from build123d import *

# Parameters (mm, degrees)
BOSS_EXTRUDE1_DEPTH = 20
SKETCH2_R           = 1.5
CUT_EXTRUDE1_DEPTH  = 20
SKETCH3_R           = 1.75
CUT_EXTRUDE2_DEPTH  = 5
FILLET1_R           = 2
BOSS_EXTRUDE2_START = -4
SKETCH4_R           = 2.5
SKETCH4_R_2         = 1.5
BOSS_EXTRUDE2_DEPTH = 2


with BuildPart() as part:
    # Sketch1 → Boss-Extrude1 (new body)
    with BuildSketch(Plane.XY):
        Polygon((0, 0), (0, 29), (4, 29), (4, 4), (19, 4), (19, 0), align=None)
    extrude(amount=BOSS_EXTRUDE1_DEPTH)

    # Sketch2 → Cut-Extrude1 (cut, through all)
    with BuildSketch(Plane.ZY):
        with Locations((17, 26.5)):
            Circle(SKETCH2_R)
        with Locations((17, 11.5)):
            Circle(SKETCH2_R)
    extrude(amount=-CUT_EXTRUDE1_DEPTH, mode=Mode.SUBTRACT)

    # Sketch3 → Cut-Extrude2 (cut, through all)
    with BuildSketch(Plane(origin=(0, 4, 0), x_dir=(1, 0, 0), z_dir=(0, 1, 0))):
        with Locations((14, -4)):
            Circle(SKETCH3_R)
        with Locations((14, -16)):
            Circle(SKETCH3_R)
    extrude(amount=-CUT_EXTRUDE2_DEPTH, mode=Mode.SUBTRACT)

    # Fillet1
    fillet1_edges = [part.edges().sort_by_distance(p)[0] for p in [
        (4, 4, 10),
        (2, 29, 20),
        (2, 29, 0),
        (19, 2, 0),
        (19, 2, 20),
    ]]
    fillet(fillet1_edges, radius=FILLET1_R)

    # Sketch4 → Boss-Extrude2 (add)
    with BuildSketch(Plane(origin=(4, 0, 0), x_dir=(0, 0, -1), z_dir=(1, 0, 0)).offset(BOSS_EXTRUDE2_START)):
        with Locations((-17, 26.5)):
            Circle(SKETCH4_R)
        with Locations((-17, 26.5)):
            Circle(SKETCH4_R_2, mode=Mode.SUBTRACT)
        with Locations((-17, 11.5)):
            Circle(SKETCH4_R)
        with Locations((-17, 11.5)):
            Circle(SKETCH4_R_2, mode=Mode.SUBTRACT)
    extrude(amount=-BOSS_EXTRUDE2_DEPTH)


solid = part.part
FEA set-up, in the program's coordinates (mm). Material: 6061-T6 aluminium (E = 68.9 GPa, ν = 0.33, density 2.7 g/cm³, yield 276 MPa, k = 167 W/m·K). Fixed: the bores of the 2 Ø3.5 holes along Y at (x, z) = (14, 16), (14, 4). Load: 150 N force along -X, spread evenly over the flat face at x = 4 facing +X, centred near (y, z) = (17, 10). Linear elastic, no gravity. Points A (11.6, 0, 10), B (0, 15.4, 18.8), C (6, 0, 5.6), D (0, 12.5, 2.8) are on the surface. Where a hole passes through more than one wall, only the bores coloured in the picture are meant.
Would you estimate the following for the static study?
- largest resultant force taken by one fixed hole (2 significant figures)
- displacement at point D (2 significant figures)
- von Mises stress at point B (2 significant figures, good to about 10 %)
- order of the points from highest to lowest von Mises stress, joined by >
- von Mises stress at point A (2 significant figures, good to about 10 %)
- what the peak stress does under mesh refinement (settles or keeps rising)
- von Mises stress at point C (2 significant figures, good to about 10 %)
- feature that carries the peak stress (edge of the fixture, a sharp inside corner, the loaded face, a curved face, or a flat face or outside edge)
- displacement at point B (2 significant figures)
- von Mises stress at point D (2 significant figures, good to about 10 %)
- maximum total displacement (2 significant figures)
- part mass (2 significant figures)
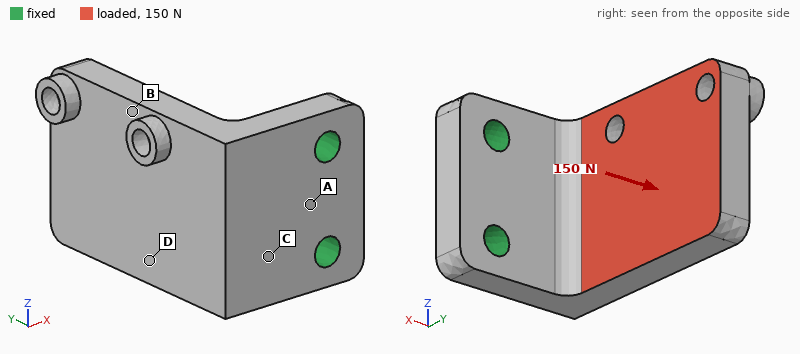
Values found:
82 N
0.050 mm
11 MPa
C > A > D > B
26 MPa
keeps rising
36 MPa
edge of the fixture
0.061 mm
17 MPa
0.13 mm
9.3 g
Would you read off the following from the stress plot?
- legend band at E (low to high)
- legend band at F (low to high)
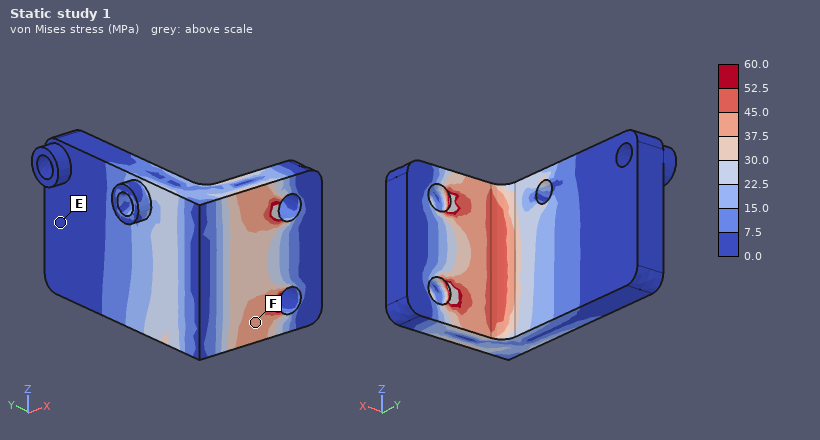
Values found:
0.0 to 7.5 MPa
37.5 to 45.0 MPa
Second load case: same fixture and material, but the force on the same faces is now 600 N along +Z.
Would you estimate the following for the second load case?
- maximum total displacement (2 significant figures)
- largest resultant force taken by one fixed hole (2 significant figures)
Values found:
0.15 mm
800 N
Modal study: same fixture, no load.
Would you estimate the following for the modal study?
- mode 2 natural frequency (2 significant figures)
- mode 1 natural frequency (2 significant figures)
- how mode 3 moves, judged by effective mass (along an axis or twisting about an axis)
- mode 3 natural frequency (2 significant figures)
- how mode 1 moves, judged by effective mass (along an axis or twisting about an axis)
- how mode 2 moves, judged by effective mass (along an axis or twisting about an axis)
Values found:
5400 Hz
2900 Hz
along Y
11 kHz
along X
along Z
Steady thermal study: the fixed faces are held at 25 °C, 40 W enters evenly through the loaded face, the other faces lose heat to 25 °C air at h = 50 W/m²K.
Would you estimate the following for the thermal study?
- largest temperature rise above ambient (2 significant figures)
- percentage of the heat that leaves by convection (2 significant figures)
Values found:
69 K
8.2 %
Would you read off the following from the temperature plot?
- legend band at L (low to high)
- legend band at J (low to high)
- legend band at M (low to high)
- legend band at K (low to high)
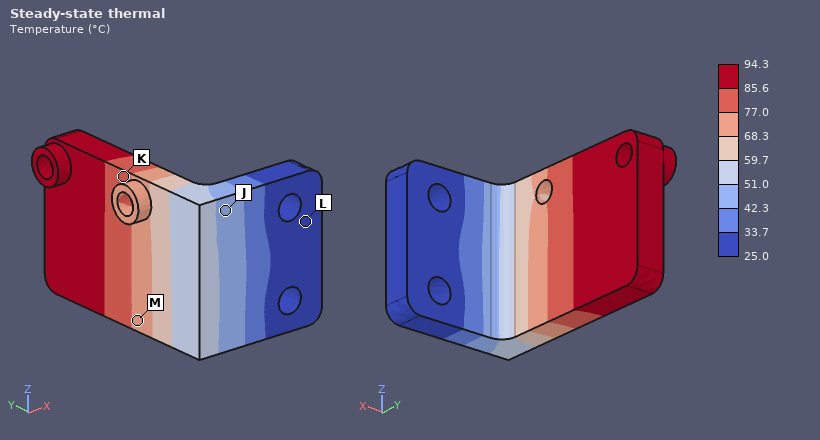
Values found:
25.0 to 33.7 °C
42.3 to 51.0 °C
68.3 to 77.0 °C
77.0 to 85.6 °C
